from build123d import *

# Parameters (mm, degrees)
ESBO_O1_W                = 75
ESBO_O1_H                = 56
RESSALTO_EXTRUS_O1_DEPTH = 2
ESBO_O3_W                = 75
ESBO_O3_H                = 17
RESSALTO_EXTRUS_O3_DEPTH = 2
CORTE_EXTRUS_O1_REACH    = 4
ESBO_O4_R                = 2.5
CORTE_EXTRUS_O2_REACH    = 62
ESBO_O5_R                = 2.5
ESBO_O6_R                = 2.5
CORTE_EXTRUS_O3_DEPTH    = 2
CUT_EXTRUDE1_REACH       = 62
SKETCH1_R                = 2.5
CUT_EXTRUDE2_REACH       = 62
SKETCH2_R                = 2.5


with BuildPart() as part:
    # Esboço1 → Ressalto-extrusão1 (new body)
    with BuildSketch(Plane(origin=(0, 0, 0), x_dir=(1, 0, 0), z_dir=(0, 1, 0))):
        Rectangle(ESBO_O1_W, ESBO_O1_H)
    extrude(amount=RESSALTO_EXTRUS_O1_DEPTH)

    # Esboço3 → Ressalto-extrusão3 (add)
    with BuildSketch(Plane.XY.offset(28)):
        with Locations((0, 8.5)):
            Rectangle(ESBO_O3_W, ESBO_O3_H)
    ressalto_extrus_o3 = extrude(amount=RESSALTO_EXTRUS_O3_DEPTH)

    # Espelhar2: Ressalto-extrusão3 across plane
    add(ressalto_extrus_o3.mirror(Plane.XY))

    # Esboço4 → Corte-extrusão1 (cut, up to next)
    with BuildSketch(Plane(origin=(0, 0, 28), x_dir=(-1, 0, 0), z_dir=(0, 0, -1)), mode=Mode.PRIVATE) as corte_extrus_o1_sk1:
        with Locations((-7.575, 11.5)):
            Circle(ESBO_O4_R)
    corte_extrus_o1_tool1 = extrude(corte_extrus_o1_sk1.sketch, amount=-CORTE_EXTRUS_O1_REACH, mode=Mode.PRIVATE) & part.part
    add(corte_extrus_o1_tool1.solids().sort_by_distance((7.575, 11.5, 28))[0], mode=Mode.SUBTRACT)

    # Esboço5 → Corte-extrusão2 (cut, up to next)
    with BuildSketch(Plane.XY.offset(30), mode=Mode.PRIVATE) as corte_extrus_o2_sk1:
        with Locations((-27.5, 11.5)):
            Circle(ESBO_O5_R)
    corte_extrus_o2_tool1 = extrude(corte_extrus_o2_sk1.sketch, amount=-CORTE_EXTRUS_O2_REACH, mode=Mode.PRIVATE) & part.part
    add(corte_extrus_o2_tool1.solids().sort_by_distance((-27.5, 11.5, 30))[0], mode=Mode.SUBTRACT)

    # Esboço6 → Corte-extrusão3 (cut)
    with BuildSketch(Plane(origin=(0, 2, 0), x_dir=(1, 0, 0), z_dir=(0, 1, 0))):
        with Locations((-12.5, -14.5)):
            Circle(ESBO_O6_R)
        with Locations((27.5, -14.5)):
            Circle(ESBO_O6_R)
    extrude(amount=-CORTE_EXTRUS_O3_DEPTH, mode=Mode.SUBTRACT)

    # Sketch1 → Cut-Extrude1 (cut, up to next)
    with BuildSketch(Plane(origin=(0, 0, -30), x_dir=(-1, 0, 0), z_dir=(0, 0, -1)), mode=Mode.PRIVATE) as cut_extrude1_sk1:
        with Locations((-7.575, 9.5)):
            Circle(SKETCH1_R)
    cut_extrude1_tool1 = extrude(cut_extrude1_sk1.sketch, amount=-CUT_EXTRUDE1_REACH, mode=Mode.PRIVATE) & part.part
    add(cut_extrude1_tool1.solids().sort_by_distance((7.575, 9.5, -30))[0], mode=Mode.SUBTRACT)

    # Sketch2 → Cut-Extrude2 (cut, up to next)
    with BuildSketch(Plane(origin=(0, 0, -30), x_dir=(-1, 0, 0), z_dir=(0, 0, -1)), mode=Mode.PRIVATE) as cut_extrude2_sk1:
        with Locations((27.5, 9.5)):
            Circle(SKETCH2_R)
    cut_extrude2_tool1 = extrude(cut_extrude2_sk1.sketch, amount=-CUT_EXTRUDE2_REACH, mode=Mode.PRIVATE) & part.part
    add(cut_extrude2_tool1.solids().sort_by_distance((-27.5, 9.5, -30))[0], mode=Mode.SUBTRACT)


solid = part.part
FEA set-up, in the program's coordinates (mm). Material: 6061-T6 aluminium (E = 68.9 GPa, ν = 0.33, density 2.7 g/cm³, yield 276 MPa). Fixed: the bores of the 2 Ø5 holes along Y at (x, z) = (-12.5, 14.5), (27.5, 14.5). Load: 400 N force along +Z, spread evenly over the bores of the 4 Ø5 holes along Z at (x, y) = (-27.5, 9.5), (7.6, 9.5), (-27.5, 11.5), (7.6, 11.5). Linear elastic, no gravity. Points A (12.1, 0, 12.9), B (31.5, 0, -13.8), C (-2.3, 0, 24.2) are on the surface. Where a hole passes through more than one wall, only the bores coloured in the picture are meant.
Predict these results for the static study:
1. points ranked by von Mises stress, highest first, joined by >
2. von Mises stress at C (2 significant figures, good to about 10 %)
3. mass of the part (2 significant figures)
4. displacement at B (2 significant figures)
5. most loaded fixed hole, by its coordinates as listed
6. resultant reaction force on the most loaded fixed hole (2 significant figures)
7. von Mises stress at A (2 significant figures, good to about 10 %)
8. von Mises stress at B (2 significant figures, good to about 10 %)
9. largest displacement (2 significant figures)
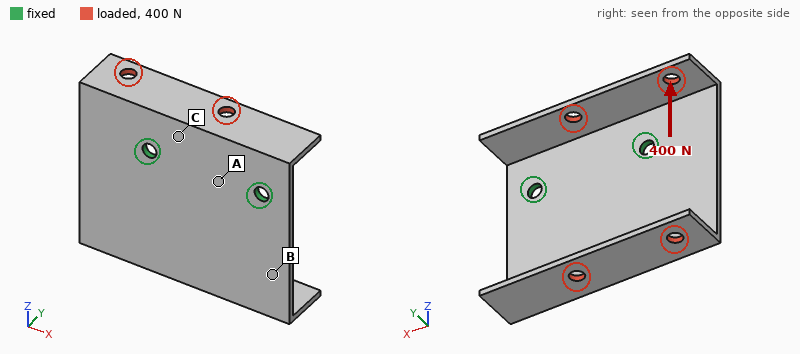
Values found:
C > B > A
44 MPa
36 g
0.18 mm
(-12.5, 14.5)
360 N
11 MPa
28 MPa
0.77 mm
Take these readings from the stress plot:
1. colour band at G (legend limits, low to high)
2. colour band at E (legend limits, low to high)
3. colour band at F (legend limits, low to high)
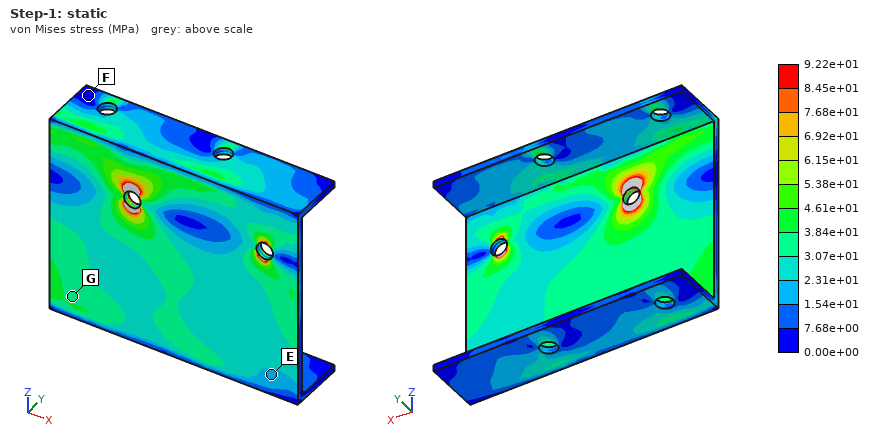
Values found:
3.07e+01 to 3.84e+01 MPa
1.54e+01 to 2.31e+01 MPa
0.00e+00 to 7.68e+00 MPa
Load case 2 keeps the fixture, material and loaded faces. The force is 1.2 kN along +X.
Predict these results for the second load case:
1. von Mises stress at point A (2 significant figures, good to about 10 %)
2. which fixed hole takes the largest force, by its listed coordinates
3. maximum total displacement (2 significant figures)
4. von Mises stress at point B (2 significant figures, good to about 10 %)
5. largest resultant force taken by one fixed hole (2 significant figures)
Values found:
24 MPa
(-12.5, 14.5)
0.98 mm
57 MPa
810 N
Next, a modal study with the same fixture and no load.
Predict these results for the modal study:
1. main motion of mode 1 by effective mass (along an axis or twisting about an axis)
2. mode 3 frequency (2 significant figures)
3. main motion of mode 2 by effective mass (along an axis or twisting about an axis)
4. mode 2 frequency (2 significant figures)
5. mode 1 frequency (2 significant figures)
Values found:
along Y
2300 Hz
twisting about Z
960 Hz
530 Hz
